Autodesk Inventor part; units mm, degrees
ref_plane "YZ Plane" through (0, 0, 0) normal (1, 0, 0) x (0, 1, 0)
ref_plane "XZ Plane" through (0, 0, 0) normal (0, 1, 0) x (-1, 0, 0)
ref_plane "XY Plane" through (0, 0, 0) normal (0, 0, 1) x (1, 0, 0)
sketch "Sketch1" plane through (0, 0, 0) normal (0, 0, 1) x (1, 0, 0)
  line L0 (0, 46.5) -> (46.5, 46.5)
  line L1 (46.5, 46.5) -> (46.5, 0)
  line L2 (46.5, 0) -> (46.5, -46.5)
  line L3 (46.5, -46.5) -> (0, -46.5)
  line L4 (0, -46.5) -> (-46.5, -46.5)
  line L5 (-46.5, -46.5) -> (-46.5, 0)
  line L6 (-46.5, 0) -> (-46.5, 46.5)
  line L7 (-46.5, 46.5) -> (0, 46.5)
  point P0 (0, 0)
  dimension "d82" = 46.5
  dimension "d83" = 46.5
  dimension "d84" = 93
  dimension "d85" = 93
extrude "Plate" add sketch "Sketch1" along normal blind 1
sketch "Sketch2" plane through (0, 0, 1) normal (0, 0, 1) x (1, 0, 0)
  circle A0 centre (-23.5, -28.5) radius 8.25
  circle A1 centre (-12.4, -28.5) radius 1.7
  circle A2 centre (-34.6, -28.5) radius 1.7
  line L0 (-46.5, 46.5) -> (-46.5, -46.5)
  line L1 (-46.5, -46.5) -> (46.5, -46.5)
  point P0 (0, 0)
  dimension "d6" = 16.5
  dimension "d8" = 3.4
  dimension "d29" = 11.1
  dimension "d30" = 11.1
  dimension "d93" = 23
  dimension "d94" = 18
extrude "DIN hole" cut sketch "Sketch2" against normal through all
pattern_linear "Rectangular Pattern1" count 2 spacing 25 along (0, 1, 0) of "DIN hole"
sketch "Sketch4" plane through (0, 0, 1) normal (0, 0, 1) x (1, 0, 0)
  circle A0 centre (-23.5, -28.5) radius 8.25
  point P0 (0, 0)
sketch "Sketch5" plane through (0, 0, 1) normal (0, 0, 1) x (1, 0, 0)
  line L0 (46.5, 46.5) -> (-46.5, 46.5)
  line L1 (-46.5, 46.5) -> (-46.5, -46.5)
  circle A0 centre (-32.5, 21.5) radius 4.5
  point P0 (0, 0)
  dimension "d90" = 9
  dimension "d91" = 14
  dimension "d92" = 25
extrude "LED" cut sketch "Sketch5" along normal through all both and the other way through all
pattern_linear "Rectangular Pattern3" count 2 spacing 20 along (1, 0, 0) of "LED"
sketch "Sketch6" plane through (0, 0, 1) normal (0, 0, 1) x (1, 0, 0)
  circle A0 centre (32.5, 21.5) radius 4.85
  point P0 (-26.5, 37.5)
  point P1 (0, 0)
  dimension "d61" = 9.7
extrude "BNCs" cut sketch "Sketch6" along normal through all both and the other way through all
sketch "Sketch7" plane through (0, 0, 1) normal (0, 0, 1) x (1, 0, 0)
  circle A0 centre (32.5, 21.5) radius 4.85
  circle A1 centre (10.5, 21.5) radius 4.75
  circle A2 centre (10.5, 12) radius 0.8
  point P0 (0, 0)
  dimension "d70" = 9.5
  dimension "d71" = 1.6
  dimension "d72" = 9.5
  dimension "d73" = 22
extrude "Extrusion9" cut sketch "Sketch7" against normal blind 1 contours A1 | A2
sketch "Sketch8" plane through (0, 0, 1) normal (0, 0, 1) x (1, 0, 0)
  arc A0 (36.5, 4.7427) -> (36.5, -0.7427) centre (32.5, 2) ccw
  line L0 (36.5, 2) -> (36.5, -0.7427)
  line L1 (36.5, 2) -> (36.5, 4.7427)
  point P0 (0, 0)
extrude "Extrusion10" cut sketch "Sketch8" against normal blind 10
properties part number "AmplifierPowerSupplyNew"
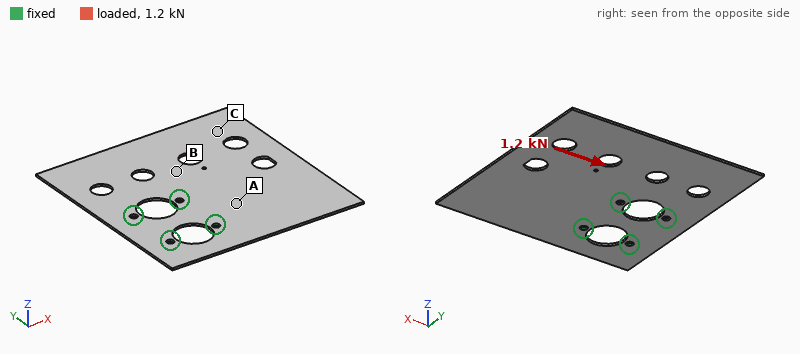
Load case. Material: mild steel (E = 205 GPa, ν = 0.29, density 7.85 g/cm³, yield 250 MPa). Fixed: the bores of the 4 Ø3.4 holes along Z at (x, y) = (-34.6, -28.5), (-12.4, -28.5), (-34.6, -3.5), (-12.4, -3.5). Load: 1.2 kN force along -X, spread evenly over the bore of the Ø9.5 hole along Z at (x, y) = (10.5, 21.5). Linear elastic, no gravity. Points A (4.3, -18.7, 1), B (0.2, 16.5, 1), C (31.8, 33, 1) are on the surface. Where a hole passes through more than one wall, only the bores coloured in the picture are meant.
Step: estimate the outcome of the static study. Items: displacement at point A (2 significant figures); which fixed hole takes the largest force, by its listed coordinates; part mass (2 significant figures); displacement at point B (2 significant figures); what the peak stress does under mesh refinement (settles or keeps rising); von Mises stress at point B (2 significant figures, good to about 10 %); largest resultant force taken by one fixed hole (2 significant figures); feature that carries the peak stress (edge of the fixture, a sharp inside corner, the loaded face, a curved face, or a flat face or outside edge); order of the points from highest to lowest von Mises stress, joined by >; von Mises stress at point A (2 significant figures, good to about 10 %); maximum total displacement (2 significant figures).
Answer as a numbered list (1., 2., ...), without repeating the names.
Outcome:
1. 5.6 µm
2. (-12.4, -3.5)
3. 62 g
4. 17 µm
5. keeps rising
6. 45 MPa
7. 1.2 kN
8. edge of the fixture
9. B > A > C
10. 23 MPa
11. 35 µm
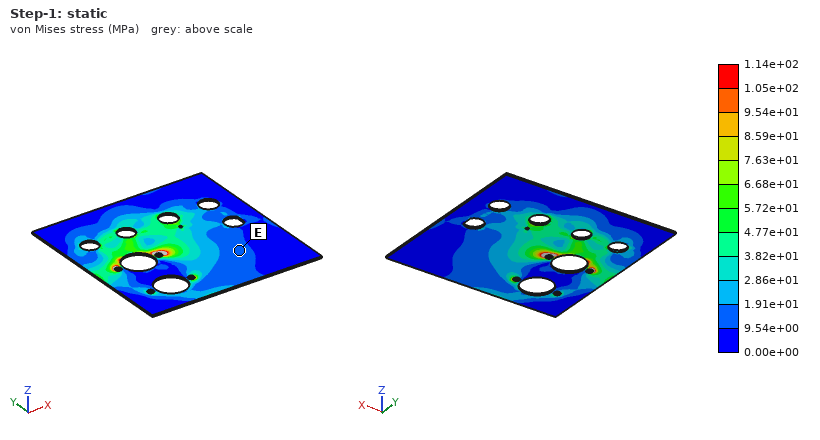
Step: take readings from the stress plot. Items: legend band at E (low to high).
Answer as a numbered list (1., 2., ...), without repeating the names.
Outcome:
1. 9.54e+00 to 1.91e+01 MPa
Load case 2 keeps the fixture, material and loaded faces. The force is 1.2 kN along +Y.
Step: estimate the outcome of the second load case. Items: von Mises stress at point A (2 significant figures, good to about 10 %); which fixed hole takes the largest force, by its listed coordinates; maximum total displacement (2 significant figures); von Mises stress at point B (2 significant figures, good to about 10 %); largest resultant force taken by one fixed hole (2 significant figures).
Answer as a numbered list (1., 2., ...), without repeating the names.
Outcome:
1. 36 MPa
2. (-12.4, -3.5)
3. 27 µm
4. 36 MPa
5. 1.1 kN
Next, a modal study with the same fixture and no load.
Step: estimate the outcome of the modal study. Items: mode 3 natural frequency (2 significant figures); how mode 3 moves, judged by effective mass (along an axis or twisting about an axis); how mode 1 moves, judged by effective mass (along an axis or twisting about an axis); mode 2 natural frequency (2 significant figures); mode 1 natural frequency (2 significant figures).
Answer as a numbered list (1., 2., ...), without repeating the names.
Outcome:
1. 440 Hz
2. along Z
3. along Z
4. 280 Hz
5. 200 Hz
